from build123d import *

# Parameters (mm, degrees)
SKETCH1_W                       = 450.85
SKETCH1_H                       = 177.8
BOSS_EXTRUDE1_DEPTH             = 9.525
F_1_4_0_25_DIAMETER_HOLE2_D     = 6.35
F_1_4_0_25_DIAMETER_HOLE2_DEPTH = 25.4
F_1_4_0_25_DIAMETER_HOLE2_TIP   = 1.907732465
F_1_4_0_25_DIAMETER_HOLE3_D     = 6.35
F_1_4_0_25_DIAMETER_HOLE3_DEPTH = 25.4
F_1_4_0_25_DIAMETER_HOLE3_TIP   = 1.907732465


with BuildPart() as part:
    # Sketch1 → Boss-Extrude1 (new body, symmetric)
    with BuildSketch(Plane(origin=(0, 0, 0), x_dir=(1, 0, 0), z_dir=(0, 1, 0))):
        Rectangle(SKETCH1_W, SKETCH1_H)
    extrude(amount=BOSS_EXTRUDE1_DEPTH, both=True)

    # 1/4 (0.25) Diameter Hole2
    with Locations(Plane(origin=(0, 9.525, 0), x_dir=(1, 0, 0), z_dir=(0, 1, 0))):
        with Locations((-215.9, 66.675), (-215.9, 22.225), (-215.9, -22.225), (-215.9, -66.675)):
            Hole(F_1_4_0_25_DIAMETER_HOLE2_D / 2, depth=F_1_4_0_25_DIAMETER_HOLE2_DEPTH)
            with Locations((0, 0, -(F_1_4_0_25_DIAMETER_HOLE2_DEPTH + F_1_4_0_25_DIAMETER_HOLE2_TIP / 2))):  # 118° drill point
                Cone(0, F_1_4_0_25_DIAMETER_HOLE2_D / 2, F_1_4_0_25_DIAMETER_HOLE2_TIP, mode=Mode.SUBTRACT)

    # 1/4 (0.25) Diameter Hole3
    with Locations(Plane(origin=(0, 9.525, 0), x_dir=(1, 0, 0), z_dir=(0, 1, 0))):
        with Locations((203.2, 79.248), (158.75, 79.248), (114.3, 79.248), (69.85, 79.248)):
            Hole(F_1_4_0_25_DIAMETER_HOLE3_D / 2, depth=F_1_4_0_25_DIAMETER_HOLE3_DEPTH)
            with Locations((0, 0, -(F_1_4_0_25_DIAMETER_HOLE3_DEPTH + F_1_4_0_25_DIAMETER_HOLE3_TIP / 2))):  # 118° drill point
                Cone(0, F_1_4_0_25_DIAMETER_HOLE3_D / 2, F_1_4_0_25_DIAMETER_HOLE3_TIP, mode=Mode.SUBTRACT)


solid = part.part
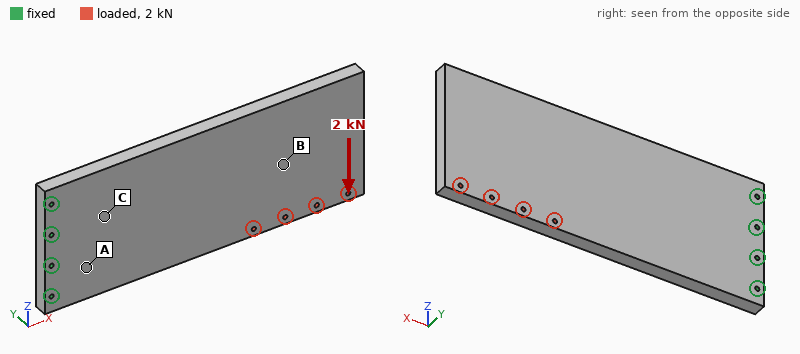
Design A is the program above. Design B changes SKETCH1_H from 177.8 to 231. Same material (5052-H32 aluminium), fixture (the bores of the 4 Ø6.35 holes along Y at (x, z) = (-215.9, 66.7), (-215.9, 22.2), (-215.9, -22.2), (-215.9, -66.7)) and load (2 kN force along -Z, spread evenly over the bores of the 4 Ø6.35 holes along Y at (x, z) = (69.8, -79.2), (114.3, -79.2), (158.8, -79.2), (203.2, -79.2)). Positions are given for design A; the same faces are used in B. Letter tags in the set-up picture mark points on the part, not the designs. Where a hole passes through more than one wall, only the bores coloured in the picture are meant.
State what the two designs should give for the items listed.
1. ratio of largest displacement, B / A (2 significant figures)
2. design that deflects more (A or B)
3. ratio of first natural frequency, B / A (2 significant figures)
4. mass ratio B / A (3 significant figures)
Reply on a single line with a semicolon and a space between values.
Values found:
0.73; A; 0.98; 1.30
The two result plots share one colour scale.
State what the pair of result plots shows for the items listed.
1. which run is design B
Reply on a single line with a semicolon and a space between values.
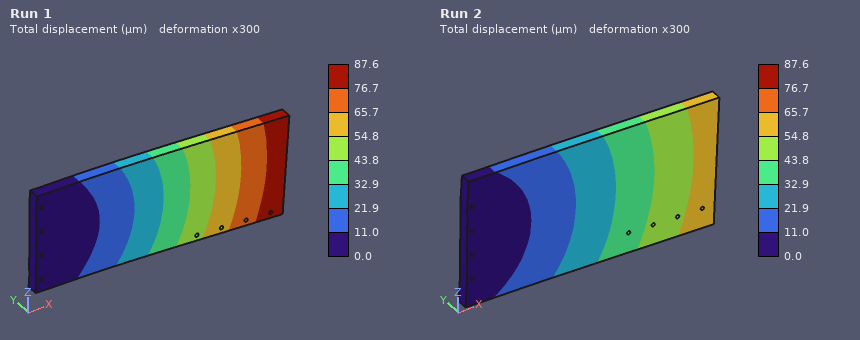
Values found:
Run 2
